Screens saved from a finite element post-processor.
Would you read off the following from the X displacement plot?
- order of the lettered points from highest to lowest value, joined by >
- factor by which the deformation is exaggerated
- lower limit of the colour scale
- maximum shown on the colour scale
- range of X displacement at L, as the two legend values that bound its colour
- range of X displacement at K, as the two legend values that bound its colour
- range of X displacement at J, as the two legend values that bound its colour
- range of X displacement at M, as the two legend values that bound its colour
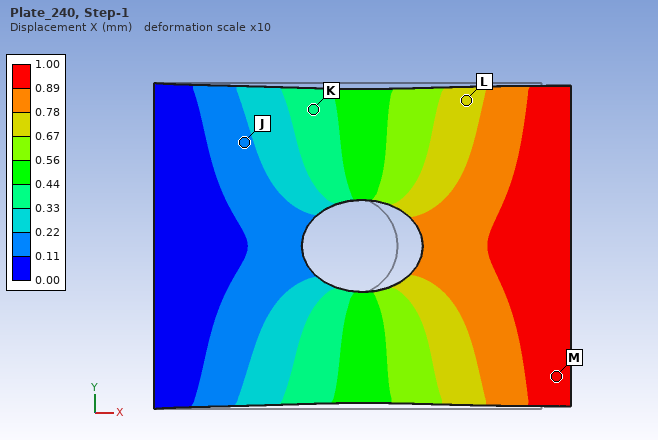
M > L > K > J
10
0.00 mm
1.00 mm
0.67 to 0.78 mm
0.33 to 0.44 mm
0.11 to 0.22 mm
0.89 to 1.00 mm
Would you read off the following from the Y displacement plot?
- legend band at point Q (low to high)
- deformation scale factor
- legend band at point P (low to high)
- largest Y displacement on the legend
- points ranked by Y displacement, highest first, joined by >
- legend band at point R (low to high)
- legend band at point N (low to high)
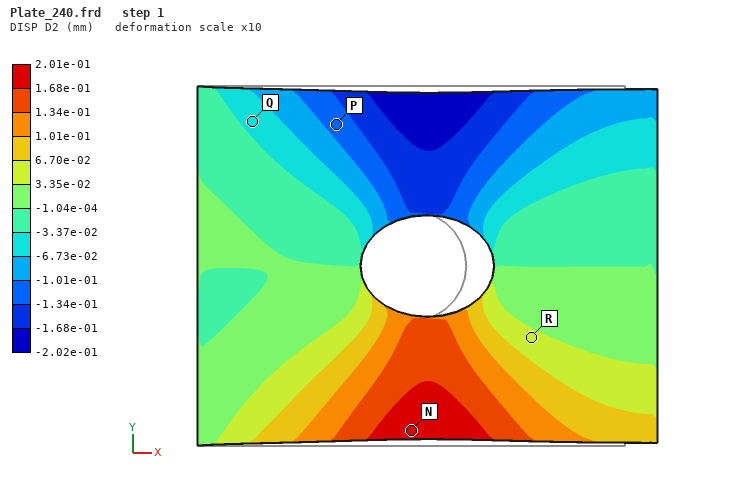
-6.73e-02 to -3.37e-02 mm
10
-1.34e-01 to -1.01e-01 mm
2.01e-01 mm
N > R > Q > P
3.35e-02 to 6.70e-02 mm
1.68e-01 to 2.01e-01 mm
